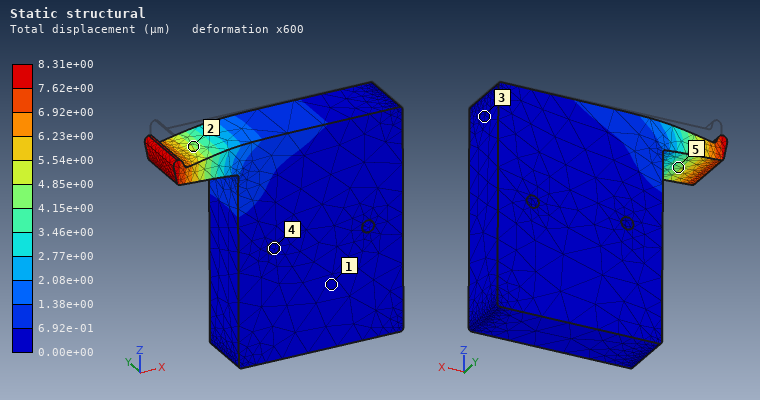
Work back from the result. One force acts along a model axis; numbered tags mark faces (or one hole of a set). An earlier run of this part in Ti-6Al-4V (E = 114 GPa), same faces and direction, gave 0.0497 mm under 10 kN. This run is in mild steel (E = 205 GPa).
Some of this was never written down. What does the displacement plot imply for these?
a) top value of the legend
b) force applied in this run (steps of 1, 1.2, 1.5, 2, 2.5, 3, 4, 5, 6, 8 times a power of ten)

8.31e+00 µm
3 kN
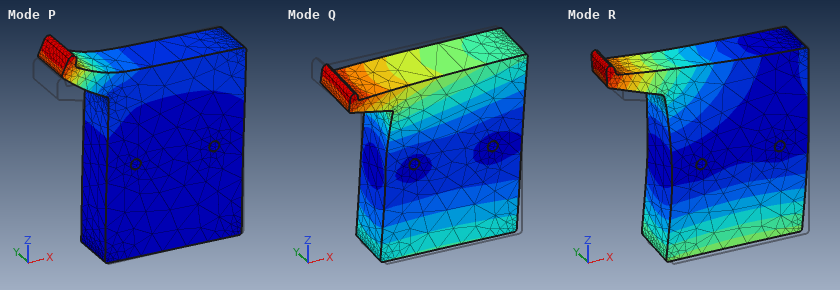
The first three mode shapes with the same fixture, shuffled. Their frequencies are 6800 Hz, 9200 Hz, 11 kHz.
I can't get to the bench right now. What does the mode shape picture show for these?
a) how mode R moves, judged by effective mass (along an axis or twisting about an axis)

along Y
